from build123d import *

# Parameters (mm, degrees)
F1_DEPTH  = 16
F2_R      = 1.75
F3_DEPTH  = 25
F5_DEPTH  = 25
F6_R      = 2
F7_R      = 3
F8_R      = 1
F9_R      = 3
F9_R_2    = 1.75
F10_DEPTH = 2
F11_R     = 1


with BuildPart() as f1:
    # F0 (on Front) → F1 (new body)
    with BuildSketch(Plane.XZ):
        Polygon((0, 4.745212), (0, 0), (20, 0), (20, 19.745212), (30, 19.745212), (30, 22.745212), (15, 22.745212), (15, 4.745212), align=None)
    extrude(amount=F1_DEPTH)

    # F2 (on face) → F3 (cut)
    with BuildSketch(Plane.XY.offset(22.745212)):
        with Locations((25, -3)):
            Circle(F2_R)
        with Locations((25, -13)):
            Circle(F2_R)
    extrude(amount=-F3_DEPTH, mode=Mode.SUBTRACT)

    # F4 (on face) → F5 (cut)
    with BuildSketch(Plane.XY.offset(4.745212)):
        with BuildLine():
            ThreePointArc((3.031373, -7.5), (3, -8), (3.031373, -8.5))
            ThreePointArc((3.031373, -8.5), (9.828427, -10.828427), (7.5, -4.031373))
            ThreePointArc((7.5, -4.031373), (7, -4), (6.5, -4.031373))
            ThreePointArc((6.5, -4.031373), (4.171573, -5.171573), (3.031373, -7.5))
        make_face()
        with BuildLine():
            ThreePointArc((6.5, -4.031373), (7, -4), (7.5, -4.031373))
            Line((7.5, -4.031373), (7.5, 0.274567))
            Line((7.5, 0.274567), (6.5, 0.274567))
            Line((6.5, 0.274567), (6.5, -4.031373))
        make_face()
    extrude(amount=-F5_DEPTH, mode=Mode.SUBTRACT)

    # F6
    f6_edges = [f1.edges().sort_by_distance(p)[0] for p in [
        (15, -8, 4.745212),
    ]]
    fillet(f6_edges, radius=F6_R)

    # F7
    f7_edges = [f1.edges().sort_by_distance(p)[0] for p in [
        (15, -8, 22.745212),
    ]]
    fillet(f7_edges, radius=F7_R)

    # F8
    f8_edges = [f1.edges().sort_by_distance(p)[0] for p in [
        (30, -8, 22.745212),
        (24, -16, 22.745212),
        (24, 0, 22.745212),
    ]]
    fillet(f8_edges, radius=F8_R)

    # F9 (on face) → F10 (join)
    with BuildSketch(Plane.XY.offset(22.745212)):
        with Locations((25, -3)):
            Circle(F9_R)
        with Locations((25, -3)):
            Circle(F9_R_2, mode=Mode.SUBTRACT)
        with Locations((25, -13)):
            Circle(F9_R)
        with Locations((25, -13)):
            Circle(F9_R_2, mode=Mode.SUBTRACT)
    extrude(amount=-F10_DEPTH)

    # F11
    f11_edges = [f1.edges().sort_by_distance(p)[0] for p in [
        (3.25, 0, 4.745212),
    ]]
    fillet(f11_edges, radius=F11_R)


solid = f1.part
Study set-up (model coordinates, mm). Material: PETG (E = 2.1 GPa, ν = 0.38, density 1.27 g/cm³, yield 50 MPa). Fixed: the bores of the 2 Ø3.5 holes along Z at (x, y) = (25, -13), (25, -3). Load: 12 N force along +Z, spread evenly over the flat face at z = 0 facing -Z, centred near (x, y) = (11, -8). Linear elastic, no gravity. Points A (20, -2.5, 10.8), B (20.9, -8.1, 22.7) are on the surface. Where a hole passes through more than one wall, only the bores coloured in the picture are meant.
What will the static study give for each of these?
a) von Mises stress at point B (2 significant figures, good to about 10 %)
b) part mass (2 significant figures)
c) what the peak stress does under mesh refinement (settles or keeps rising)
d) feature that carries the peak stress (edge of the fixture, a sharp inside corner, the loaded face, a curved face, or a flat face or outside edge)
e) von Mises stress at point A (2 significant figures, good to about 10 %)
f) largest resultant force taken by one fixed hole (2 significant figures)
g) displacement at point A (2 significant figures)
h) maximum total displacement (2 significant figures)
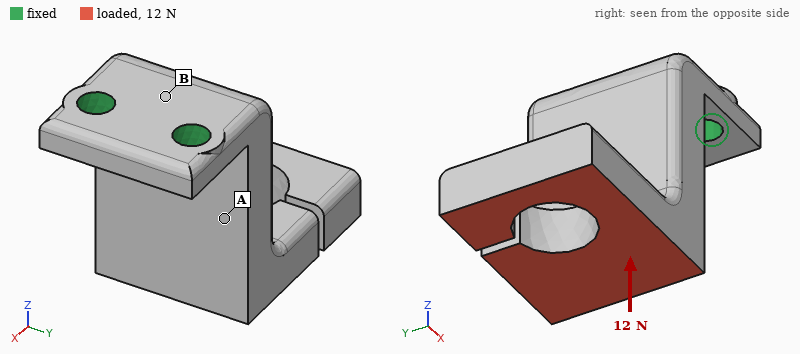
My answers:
3.8 MPa
3.9 g
keeps rising
edge of the fixture
1.1 MPa
6.2 N
0.10 mm
0.44 mm
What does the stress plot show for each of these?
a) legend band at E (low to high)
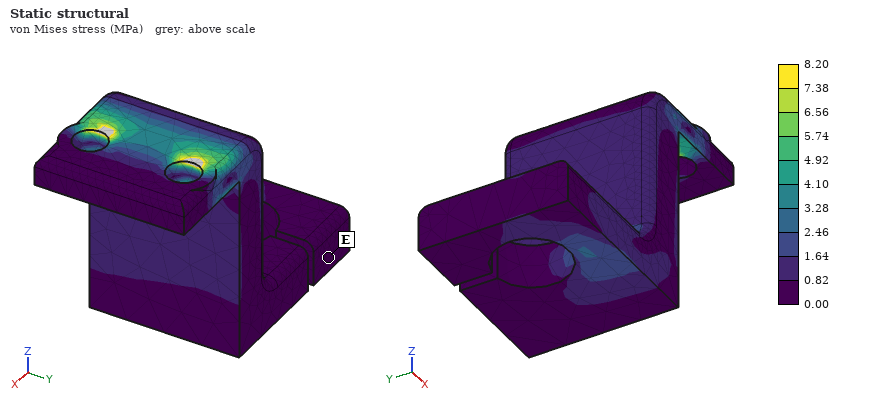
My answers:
0.00 to 0.82 MPa
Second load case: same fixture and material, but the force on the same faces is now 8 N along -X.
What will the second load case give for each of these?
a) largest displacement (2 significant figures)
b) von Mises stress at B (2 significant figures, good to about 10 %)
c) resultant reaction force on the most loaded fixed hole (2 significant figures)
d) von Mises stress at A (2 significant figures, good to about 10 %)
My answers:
0.48 mm
5.3 MPa
4.9 N
1.3 MPa
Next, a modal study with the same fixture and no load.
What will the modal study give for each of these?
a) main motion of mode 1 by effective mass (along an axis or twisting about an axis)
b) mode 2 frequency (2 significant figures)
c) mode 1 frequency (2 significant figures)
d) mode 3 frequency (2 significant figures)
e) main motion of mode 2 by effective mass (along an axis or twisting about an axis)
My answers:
along X
1300 Hz
550 Hz
1700 Hz
along Y
